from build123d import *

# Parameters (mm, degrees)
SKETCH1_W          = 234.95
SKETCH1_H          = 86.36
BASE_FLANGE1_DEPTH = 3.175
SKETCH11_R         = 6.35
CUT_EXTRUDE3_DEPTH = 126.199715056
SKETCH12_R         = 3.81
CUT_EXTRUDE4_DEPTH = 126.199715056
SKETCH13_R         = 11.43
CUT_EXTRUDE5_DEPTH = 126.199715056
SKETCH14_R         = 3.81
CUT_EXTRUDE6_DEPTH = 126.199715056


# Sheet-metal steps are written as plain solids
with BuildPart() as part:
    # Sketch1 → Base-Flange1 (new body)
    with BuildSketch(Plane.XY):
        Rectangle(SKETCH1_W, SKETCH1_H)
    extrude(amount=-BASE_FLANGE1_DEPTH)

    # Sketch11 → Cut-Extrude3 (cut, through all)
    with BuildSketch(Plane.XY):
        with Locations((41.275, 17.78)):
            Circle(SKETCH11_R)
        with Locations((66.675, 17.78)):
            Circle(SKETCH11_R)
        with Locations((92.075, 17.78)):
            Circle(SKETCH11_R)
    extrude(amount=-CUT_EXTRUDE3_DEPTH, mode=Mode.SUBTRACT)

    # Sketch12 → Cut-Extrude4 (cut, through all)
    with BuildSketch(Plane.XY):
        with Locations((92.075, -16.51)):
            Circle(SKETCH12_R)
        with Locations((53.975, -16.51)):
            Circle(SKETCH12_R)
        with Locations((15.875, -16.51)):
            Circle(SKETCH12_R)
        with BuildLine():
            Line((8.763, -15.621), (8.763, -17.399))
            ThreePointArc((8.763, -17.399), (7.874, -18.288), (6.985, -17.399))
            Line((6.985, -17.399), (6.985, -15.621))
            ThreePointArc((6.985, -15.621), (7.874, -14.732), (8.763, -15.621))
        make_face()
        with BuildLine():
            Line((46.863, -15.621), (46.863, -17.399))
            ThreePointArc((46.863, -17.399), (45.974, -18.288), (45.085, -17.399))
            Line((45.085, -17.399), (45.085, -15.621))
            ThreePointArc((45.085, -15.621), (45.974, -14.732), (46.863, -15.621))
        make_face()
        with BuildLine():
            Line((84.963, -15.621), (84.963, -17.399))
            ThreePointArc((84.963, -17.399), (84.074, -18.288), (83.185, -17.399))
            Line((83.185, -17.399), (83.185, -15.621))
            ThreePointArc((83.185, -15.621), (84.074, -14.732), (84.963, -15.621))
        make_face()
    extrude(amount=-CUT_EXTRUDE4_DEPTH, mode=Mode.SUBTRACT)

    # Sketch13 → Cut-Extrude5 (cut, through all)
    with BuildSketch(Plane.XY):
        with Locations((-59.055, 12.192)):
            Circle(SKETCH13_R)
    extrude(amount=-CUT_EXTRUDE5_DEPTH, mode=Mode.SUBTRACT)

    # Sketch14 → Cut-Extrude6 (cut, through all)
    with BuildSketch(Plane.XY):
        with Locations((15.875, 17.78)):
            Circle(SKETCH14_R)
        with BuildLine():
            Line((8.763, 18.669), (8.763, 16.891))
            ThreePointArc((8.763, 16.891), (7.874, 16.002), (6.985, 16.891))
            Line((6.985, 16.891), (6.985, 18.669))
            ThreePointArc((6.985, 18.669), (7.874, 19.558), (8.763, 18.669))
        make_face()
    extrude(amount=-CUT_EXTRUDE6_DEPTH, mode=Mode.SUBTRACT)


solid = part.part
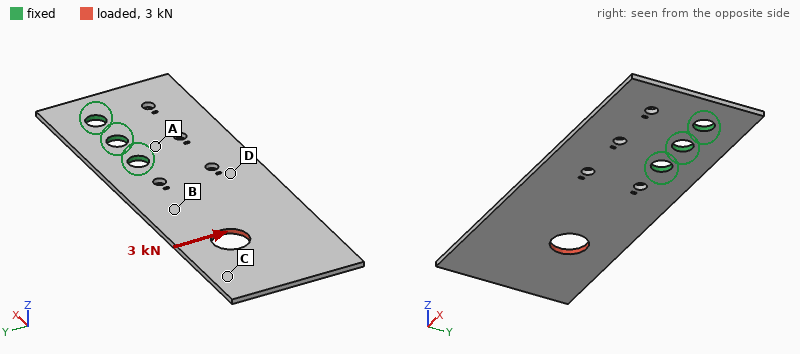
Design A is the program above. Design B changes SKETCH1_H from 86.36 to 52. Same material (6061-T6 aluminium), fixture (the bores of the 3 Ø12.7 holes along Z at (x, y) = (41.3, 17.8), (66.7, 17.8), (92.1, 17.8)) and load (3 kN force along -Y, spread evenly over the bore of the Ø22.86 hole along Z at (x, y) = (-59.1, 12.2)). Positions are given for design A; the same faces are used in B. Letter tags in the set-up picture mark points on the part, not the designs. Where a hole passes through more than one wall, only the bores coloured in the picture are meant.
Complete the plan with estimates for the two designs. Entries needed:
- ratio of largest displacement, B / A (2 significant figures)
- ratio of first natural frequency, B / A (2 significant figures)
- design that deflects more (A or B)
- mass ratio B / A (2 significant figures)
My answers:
2.9
1.0
B
0.58
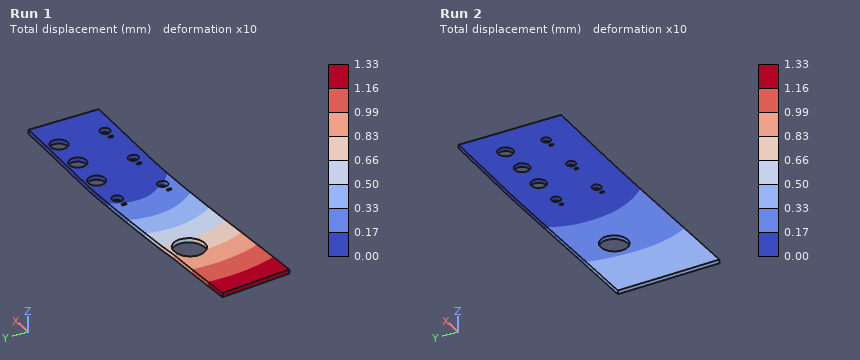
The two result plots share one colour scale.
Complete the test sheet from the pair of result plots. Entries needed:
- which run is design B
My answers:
Run 1
